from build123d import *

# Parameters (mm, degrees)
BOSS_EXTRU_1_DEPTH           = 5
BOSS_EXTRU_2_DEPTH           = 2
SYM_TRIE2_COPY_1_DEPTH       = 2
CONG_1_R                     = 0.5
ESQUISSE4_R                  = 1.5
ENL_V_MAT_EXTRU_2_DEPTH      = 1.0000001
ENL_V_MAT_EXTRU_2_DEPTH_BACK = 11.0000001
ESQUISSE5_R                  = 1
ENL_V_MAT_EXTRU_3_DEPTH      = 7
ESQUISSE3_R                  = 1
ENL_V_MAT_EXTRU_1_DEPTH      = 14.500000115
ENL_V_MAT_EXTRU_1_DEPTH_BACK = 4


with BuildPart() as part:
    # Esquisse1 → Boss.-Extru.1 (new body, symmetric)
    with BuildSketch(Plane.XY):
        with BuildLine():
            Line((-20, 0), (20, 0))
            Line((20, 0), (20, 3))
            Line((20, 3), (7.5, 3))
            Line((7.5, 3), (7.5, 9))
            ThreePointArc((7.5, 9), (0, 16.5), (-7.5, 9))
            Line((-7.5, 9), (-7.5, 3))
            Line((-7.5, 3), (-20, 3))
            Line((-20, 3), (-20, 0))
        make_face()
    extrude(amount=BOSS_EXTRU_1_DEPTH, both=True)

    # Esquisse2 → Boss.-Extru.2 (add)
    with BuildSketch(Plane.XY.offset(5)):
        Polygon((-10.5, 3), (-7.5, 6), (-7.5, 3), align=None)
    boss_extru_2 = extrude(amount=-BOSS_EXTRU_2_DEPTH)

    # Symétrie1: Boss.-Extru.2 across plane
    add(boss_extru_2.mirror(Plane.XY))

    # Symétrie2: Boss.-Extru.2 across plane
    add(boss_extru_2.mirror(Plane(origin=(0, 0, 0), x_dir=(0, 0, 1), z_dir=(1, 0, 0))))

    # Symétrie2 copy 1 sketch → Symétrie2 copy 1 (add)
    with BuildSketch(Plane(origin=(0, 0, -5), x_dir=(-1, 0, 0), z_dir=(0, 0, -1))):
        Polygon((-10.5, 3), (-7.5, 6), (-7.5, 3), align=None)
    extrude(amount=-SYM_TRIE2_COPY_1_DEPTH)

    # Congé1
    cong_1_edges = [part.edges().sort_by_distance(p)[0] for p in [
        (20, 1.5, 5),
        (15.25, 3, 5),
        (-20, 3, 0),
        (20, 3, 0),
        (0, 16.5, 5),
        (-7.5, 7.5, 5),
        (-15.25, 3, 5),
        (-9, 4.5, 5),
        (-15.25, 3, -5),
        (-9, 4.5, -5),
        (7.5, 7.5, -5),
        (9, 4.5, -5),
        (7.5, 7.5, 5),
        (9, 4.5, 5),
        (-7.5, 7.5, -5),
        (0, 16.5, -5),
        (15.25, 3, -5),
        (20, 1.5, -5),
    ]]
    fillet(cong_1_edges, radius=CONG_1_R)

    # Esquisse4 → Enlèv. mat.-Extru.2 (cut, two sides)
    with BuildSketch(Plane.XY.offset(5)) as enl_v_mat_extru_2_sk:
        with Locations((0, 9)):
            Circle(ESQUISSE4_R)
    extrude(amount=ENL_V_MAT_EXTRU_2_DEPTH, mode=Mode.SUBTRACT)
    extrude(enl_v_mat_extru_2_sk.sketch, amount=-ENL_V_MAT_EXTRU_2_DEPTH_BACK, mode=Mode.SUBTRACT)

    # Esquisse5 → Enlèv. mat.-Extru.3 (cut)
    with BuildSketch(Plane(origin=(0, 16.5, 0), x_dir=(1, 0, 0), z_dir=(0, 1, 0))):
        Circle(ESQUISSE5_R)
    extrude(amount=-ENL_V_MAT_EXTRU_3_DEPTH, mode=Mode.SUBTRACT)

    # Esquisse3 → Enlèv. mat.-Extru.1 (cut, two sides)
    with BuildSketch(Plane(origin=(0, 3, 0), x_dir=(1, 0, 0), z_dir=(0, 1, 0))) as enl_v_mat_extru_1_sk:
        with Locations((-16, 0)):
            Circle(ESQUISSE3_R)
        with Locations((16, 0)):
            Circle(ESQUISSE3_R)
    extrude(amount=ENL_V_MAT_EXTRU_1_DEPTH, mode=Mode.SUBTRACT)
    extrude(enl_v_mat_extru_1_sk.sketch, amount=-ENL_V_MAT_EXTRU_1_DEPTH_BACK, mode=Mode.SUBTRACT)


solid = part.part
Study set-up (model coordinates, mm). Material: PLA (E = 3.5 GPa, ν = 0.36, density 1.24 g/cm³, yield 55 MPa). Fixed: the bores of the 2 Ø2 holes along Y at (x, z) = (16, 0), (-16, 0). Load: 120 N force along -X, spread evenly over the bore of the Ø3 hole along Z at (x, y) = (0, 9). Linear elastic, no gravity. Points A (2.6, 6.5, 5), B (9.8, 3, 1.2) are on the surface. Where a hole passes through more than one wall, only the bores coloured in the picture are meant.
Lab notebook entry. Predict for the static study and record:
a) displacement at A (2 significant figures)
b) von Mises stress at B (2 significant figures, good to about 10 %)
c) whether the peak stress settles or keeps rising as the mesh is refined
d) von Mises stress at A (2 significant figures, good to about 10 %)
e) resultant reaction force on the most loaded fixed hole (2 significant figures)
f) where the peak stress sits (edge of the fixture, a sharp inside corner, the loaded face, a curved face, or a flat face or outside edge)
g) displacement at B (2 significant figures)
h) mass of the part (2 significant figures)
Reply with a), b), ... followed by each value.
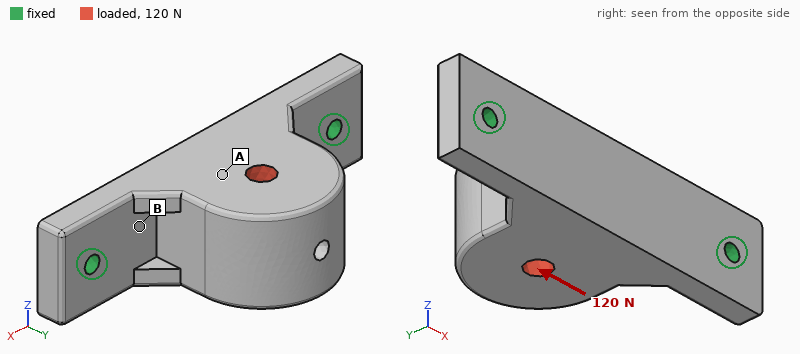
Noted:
a) 22 µm
b) 6.5 MPa
c) keeps rising
d) 1.6 MPa
e) 70 N
f) edge of the fixture
g) 18 µm
h) 3.6 g
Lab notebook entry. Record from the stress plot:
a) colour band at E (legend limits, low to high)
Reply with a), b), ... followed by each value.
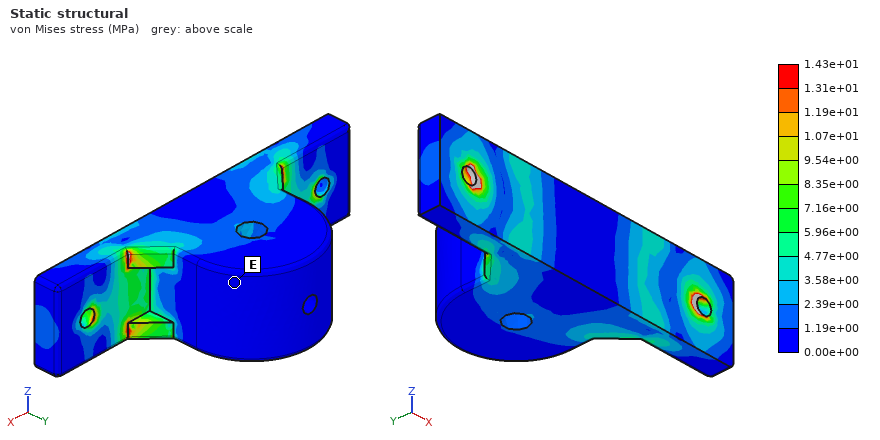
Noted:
a) 0.00e+00 to 1.19e+00 MPa
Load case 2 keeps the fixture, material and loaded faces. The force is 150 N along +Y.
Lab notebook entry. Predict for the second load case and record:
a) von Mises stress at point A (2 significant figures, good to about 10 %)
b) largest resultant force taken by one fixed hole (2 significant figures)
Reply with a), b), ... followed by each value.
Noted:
a) 3.1 MPa
b) 88 N
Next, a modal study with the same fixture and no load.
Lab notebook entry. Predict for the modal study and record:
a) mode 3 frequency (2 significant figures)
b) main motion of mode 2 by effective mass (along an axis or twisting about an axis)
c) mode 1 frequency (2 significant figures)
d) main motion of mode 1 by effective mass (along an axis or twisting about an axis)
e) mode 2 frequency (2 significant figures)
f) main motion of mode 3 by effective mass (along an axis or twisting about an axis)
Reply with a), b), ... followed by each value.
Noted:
a) 5600 Hz
b) along Y
c) 1900 Hz
d) along Z
e) 3900 Hz
f) along X
